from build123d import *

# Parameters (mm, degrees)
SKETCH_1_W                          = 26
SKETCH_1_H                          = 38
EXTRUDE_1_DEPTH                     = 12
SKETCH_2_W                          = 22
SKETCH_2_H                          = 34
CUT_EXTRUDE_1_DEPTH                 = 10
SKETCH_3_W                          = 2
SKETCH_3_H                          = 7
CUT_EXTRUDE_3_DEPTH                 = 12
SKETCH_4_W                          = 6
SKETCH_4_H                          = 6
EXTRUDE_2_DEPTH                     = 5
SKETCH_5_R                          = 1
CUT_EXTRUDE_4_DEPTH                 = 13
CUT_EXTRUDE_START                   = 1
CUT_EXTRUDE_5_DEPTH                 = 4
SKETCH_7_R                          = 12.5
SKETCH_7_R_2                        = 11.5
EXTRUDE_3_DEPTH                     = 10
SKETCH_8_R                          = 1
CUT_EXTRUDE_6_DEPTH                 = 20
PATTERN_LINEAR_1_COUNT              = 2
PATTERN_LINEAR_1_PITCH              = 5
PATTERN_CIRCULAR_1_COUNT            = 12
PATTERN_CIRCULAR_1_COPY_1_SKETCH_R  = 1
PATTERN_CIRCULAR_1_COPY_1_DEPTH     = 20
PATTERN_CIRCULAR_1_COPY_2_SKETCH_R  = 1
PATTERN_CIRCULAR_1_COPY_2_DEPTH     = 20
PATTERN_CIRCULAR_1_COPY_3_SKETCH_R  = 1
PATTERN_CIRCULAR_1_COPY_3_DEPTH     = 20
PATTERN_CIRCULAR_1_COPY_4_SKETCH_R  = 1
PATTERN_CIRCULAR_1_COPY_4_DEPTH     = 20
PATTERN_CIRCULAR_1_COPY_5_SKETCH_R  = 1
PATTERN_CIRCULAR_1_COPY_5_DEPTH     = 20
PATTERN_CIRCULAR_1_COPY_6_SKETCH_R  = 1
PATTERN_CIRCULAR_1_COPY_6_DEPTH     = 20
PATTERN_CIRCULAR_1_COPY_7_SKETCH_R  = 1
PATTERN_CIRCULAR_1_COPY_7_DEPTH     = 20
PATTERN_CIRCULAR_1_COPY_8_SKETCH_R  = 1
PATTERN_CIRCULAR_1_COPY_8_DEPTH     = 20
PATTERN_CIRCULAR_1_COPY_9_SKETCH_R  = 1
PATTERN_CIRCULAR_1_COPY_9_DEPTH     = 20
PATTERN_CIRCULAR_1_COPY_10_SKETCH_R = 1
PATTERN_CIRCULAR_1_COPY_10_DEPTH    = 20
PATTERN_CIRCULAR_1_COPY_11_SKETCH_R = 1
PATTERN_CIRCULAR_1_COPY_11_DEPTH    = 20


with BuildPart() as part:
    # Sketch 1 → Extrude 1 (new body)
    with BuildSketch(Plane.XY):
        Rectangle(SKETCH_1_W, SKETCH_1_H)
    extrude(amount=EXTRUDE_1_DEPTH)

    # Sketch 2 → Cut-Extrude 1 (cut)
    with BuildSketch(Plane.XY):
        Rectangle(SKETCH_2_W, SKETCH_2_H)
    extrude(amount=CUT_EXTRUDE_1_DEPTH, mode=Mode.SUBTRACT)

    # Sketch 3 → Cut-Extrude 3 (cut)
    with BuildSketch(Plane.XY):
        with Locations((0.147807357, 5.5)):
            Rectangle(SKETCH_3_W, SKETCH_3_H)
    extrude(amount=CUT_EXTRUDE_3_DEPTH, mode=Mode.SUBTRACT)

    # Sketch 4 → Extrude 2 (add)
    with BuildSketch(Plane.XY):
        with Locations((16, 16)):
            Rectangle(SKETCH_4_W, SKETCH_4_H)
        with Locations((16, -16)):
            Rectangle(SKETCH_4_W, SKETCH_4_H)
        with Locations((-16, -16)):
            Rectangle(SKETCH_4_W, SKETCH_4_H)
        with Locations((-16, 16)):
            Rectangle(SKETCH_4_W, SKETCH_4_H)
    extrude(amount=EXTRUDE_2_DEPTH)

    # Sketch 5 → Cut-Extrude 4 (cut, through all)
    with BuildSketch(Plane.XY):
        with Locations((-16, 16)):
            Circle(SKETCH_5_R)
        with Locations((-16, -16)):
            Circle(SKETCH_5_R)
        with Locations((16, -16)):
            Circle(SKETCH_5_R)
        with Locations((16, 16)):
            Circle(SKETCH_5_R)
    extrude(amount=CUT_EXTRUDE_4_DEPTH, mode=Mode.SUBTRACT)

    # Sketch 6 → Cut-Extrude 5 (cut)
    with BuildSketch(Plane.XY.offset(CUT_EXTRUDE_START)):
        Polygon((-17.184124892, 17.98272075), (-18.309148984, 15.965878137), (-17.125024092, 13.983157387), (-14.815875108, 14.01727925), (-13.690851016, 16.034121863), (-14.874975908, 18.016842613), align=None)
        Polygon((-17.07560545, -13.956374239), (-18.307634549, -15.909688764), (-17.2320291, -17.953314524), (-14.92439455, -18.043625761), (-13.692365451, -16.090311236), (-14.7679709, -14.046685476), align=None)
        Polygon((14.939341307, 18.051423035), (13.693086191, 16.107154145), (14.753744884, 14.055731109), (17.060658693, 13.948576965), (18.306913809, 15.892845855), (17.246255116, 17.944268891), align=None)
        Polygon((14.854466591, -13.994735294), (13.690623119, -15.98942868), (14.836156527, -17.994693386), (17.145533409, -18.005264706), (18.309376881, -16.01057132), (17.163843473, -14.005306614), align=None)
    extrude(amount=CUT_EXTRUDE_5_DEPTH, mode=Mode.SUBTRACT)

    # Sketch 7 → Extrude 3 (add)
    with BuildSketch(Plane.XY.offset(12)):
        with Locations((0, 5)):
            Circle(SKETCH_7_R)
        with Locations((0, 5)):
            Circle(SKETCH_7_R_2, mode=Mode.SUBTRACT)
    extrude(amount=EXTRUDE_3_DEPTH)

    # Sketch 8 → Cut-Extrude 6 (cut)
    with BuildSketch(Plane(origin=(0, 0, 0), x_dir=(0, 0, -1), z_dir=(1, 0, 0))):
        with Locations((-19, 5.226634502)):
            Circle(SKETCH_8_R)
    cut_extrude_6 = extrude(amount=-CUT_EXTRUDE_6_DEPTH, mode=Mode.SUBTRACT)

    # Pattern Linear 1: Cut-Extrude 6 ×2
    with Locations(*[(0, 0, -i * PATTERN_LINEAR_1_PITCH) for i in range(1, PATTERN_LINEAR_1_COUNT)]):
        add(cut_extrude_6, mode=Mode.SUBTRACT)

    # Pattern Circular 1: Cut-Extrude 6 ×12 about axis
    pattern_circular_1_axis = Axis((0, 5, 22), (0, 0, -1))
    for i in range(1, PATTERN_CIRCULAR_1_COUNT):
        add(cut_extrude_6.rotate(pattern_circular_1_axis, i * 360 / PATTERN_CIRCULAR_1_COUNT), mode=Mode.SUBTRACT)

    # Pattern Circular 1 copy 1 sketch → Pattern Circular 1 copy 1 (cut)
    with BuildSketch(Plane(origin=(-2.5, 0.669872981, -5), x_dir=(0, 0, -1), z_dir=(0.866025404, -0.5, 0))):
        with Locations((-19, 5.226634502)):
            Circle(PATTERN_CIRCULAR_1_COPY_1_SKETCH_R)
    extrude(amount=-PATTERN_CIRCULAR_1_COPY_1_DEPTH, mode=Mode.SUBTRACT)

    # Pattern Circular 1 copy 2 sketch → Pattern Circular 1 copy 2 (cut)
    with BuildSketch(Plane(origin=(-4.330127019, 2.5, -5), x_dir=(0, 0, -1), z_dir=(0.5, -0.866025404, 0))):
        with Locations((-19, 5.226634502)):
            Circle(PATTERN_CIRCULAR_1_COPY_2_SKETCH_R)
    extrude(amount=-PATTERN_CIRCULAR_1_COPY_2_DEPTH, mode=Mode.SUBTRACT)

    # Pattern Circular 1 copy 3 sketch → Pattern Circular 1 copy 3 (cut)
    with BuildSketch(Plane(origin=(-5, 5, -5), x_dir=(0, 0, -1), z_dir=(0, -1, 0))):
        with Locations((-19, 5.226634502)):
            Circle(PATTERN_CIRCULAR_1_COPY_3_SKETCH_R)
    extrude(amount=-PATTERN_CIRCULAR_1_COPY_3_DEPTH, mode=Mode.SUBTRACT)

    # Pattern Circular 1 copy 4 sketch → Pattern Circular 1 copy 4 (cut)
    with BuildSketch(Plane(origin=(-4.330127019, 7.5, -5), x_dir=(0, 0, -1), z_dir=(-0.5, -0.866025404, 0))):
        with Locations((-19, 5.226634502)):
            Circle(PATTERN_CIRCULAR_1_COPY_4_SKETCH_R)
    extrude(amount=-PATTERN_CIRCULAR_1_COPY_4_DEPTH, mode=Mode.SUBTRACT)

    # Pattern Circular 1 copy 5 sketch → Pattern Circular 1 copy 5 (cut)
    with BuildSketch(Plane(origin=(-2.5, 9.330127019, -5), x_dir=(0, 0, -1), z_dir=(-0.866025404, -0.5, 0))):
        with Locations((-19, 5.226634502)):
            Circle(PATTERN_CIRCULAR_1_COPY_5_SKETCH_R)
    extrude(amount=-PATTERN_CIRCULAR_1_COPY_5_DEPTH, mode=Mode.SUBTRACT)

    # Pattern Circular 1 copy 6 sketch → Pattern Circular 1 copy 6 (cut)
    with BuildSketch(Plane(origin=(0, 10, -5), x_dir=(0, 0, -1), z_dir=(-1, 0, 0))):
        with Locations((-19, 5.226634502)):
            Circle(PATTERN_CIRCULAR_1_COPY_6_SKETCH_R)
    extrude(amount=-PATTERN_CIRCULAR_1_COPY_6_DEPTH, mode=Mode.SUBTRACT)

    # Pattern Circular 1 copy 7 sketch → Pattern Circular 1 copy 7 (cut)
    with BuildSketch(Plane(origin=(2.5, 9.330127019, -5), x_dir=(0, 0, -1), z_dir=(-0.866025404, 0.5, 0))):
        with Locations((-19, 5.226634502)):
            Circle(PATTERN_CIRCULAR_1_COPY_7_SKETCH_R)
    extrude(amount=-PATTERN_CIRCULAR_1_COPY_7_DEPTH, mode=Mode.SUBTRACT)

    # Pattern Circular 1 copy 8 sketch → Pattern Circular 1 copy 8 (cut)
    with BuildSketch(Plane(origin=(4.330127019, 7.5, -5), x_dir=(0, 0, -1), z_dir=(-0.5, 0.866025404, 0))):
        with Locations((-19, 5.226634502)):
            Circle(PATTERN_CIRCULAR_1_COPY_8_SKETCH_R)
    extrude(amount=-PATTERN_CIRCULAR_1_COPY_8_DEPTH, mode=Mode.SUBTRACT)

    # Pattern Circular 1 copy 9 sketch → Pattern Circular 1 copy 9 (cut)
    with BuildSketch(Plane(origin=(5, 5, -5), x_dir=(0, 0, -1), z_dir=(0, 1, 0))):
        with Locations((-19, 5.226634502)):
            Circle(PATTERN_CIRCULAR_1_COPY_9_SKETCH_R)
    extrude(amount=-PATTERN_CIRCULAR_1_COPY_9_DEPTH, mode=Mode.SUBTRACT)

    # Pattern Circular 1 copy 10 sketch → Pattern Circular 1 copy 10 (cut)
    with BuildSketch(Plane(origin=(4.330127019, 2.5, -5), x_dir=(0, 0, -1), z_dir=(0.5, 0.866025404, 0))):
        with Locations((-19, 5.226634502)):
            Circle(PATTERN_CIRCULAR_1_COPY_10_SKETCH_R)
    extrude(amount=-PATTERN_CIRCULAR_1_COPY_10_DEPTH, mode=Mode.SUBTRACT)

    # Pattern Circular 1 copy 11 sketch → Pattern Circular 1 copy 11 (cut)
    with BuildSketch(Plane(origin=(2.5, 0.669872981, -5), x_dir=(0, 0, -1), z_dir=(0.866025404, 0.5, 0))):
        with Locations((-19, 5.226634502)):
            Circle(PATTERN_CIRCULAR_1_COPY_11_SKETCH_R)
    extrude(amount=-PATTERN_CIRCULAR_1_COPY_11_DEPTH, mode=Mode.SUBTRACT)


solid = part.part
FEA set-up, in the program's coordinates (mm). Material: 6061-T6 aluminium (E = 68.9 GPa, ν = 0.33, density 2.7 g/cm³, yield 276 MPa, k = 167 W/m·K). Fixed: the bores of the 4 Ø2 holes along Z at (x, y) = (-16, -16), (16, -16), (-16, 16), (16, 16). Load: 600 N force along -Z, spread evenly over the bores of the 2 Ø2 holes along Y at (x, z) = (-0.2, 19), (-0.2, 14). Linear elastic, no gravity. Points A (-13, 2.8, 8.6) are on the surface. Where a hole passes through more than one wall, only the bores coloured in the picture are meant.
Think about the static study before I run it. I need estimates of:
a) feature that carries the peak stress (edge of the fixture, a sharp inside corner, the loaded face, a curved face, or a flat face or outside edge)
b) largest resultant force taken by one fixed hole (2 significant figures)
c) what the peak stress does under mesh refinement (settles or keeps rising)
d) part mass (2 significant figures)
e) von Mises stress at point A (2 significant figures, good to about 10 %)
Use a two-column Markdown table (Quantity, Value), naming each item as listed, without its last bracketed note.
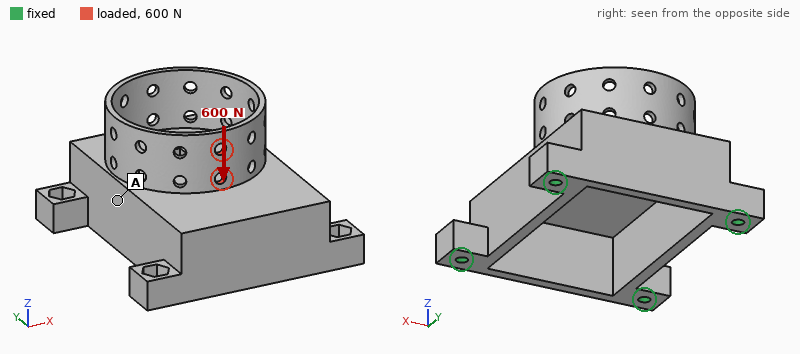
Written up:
| Quantity | Value |
|---|---|
| feature that carries the peak stress | edge of the fixture |
| largest resultant force taken by one fixed hole | 270 N |
| what the peak stress does under mesh refinement | keeps rising |
| part mass | 15 g |
| von Mises stress at point A | 15 MPa |
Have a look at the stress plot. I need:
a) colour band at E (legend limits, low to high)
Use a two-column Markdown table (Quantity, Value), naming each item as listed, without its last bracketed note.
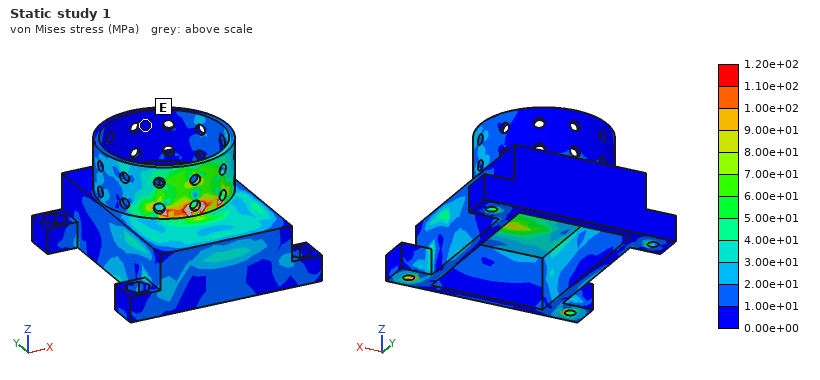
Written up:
| Quantity | Value |
|---|---|
| colour band at E | 0.00e+00 to 1.00e+01 MPa |
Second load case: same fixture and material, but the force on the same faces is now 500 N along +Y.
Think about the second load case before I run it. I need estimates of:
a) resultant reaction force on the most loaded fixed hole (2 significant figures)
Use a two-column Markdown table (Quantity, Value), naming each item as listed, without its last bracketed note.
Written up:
| Quantity | Value |
|---|---|
| resultant reaction force on the most loaded fixed hole | 180 N |
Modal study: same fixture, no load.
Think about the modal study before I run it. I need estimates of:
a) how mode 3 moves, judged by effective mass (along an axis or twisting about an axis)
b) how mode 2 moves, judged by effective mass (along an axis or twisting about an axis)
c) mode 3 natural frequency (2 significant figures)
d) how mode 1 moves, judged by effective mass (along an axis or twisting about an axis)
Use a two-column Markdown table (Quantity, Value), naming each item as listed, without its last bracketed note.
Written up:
| Quantity | Value |
|---|---|
| how mode 3 moves, judged by effective mass | along X |
| how mode 2 moves, judged by effective mass | along Z |
| mode 3 natural frequency | 15 kHz |
| how mode 1 moves, judged by effective mass | along Y |
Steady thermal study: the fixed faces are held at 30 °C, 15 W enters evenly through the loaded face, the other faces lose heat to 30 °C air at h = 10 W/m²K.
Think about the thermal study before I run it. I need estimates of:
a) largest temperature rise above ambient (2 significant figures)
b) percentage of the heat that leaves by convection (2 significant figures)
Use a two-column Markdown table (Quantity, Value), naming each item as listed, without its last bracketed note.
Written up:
| Quantity | Value |
|---|---|
| largest temperature rise above ambient | 53 K |
| percentage of the heat that leaves by convection | 5.5 % |
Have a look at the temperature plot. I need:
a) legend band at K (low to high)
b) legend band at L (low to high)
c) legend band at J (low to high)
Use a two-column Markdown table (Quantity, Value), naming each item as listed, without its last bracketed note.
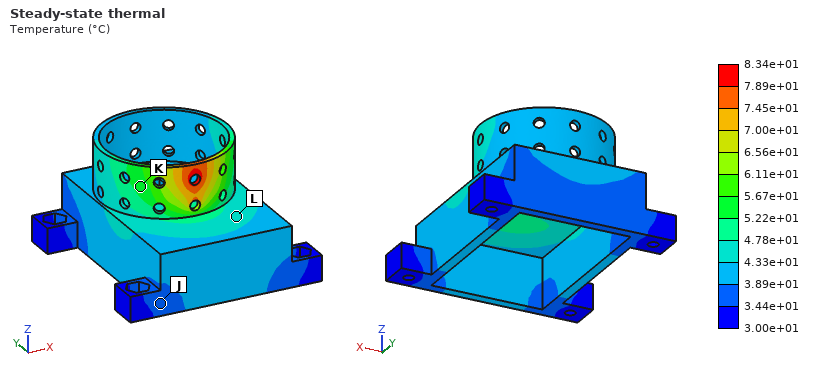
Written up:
| Quantity | Value |
|---|---|
| legend band at K | 5.22e+01 to 5.67e+01 °C |
| legend band at L | 4.33e+01 to 4.78e+01 °C |
| legend band at J | 3.44e+01 to 3.89e+01 °C |
